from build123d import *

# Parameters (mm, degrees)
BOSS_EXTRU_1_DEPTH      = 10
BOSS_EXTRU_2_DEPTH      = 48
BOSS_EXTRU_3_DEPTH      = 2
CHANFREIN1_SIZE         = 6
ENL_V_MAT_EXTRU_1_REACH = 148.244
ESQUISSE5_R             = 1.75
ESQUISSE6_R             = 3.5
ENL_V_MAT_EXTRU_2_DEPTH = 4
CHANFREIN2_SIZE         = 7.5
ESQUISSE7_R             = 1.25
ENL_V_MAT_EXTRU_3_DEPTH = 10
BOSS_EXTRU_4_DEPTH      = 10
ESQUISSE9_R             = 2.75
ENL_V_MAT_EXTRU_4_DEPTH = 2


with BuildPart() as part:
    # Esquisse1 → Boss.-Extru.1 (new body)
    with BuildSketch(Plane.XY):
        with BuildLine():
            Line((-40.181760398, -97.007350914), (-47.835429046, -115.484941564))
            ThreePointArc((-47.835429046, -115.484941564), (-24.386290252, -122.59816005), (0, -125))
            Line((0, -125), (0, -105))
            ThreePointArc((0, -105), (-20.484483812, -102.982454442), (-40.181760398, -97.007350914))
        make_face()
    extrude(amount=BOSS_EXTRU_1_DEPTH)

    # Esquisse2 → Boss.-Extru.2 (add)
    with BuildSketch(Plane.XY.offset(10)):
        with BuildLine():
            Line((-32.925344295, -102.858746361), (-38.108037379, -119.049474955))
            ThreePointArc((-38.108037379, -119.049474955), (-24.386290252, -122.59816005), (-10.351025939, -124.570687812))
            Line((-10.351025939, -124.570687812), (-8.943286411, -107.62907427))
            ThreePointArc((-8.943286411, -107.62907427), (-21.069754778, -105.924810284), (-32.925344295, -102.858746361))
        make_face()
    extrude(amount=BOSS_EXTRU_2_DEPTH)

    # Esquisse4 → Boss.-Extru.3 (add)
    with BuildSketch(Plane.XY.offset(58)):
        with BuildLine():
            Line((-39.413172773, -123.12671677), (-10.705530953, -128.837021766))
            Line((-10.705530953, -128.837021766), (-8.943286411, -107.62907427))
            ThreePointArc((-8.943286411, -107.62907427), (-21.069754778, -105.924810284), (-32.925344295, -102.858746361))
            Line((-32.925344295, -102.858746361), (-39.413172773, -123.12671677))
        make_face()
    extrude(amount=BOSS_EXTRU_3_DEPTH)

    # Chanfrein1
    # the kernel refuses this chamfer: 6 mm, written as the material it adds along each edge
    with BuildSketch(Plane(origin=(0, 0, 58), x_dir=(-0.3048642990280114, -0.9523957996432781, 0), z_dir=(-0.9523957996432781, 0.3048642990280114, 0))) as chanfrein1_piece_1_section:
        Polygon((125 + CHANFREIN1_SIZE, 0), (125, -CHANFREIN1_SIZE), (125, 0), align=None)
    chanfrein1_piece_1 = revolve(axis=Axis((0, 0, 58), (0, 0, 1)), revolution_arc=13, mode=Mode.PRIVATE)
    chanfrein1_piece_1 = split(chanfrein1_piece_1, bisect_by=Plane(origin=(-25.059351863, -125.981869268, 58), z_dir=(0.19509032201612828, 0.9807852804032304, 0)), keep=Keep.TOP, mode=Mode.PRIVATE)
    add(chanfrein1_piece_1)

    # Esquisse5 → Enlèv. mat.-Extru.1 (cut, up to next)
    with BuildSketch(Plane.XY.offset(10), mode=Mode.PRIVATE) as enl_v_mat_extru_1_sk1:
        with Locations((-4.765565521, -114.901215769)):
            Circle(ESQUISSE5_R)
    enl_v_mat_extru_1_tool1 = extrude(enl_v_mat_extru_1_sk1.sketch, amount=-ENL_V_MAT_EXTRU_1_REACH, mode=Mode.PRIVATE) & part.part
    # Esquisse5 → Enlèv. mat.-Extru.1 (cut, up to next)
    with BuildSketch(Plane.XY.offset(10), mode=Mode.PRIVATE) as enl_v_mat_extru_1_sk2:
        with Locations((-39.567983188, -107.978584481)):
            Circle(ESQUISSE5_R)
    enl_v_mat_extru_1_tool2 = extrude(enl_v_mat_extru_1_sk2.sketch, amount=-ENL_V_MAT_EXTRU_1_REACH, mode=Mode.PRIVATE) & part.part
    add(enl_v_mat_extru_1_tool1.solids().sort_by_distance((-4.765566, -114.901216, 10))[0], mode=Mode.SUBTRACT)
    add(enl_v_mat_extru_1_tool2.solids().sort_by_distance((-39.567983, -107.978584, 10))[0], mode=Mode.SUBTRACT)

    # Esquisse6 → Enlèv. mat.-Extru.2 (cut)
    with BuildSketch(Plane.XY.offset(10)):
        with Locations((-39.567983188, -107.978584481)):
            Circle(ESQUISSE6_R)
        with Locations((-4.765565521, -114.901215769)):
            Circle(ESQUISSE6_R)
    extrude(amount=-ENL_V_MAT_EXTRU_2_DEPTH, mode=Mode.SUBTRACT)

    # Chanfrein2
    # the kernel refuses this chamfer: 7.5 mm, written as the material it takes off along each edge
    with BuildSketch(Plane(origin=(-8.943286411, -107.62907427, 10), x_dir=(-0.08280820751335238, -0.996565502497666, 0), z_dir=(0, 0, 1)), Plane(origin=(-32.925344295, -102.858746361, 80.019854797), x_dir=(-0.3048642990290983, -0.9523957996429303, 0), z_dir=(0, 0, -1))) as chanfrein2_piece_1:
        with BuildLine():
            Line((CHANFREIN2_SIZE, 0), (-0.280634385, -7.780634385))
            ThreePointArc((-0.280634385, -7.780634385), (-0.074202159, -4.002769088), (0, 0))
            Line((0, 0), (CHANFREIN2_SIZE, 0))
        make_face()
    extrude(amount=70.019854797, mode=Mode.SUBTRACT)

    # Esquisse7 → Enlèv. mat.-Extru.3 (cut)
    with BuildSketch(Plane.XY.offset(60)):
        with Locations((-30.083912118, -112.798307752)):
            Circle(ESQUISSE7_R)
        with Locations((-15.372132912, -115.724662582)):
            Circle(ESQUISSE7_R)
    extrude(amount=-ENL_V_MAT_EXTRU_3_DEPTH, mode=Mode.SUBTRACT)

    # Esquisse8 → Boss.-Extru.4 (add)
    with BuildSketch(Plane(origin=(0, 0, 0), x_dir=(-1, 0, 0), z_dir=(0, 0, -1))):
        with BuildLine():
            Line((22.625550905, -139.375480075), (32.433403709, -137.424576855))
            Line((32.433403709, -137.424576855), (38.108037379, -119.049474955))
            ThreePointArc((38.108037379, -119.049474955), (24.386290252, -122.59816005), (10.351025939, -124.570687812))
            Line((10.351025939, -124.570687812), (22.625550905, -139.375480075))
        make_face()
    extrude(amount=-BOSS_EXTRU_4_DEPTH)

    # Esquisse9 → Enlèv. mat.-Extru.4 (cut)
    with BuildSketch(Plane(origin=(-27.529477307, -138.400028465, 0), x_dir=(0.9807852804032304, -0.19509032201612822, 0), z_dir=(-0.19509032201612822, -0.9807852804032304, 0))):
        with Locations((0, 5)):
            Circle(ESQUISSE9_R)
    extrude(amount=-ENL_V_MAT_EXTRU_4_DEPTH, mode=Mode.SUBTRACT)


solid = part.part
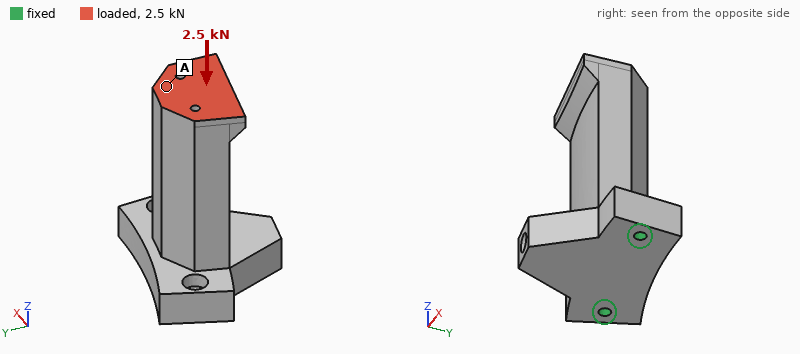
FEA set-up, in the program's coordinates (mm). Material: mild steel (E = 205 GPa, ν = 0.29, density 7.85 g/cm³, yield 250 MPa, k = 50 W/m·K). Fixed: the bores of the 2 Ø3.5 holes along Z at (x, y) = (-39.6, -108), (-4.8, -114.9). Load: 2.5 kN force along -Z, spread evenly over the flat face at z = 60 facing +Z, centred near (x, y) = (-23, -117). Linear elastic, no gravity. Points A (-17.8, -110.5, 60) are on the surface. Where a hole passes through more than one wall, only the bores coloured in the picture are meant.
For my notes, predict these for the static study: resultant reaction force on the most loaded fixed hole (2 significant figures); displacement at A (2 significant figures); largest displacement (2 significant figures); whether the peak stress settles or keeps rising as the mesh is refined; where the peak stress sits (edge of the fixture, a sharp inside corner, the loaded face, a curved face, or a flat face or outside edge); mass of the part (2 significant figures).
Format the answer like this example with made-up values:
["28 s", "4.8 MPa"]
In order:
["1.3 kN", "27 µm", "29 µm", "keeps rising", "edge of the fixture", "250 g"]
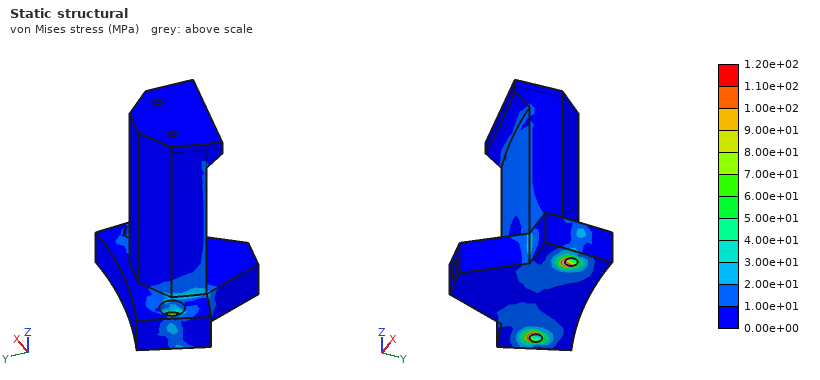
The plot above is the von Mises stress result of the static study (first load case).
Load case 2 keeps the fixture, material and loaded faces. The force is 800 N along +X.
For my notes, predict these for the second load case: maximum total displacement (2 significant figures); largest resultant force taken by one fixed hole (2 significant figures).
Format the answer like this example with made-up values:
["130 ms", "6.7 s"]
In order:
["29 µm", "1.4 kN"]
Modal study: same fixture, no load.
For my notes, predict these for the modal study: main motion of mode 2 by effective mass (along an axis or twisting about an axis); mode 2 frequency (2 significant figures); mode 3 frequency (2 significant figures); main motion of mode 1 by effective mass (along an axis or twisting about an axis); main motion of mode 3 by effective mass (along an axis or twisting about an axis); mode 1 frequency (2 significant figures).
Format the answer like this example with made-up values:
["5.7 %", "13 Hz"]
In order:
["along X", "4700 Hz", "9900 Hz", "along Y", "along Z", "1800 Hz"]
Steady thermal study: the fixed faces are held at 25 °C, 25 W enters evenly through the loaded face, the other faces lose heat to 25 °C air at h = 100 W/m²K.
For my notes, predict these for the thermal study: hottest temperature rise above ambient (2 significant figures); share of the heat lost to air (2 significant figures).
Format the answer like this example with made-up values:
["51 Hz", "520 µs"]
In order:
["53 K", "58 %"]
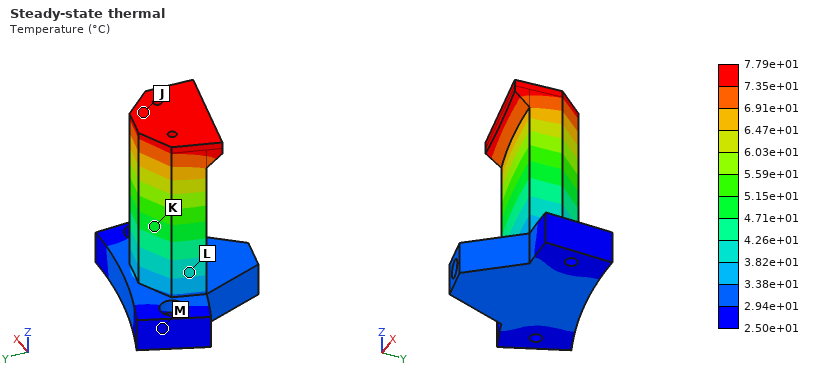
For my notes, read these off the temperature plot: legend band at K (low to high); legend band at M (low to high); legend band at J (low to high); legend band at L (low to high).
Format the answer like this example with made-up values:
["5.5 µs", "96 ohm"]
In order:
["4.71e+01 to 5.15e+01 °C", "2.50e+01 to 2.94e+01 °C", "7.35e+01 to 7.79e+01 °C", "3.82e+01 to 4.26e+01 °C"]
